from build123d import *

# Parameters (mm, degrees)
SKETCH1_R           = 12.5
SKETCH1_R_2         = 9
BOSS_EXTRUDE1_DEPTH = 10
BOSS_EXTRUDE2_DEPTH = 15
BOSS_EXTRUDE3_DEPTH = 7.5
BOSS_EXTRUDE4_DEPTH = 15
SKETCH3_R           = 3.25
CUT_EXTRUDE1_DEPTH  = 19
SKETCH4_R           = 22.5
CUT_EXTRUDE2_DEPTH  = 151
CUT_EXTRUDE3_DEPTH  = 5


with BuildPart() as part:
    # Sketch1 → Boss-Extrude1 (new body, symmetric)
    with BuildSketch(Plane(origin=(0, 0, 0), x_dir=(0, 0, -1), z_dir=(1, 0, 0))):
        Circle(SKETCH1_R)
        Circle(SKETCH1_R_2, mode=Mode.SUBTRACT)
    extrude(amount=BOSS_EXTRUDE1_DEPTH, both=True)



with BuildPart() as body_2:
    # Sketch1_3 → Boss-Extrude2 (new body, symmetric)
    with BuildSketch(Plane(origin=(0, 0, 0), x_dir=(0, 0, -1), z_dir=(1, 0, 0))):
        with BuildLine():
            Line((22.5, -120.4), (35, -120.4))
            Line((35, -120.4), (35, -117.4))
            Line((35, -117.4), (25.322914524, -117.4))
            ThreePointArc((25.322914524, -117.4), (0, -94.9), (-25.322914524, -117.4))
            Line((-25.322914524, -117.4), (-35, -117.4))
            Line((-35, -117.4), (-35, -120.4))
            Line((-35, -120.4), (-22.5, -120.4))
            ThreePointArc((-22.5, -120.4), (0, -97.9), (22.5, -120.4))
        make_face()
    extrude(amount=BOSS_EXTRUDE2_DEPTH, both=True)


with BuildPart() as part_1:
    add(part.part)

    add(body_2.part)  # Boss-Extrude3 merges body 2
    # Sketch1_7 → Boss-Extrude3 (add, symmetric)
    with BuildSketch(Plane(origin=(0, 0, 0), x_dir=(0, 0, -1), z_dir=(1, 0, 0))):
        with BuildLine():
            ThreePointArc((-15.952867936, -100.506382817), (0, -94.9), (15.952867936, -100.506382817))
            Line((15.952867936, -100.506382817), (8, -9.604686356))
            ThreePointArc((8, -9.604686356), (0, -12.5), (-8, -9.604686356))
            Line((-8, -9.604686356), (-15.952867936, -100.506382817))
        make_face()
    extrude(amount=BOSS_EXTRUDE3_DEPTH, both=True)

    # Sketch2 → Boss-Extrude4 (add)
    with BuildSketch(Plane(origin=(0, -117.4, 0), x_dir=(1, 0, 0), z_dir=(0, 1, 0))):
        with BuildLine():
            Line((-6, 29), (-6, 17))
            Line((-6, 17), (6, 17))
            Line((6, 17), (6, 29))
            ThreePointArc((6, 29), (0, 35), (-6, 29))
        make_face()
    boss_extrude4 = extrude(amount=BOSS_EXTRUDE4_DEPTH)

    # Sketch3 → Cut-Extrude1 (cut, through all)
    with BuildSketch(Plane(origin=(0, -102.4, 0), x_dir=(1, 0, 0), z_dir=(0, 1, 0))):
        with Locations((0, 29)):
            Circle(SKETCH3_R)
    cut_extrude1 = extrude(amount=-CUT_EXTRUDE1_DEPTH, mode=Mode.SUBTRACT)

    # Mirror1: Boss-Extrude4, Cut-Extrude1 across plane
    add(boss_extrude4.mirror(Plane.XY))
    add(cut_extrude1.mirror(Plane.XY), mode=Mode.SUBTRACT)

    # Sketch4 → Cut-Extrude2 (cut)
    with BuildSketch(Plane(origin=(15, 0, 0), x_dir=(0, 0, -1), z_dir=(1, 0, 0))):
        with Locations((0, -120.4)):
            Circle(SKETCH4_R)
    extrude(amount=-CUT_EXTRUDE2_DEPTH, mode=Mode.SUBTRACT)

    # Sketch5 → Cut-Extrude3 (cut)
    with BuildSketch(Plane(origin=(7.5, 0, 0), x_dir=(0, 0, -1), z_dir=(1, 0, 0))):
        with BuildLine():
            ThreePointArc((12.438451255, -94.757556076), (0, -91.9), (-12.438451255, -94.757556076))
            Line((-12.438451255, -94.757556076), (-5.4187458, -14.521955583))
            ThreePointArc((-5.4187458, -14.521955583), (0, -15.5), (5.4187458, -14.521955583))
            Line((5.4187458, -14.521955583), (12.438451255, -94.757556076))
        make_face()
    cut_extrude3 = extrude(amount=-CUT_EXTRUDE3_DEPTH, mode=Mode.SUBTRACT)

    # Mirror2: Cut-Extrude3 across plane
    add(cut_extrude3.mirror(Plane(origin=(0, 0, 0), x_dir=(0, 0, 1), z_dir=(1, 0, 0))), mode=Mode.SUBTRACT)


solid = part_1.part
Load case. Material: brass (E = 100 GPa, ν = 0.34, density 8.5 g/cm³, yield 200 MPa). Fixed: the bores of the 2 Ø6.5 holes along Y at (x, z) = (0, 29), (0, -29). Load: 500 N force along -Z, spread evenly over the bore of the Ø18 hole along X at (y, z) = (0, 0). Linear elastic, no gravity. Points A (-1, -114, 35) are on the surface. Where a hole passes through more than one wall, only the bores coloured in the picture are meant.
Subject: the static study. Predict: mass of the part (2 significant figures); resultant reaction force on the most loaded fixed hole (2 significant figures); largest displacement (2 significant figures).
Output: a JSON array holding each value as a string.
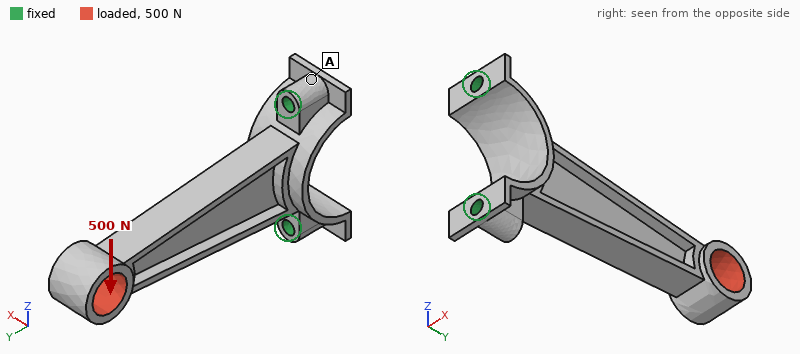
["280 g", "1.5 kN", "0.23 mm"]
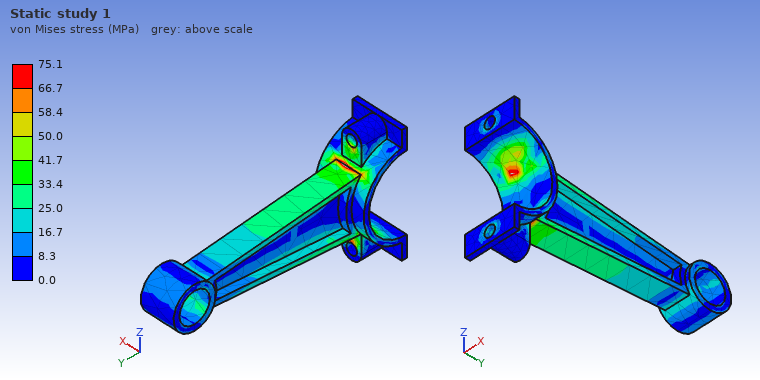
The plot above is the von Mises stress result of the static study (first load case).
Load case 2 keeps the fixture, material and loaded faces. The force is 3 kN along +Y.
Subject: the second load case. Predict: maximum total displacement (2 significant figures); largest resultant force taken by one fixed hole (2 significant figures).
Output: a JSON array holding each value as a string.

["39 µm", "1.9 kN"]
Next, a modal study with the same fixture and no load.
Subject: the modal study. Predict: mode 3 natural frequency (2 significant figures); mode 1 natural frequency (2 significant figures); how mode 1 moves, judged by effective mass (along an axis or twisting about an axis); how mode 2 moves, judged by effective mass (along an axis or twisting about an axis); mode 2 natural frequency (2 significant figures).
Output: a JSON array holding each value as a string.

["1700 Hz", "420 Hz", "along X", "along Z", "1000 Hz"]
